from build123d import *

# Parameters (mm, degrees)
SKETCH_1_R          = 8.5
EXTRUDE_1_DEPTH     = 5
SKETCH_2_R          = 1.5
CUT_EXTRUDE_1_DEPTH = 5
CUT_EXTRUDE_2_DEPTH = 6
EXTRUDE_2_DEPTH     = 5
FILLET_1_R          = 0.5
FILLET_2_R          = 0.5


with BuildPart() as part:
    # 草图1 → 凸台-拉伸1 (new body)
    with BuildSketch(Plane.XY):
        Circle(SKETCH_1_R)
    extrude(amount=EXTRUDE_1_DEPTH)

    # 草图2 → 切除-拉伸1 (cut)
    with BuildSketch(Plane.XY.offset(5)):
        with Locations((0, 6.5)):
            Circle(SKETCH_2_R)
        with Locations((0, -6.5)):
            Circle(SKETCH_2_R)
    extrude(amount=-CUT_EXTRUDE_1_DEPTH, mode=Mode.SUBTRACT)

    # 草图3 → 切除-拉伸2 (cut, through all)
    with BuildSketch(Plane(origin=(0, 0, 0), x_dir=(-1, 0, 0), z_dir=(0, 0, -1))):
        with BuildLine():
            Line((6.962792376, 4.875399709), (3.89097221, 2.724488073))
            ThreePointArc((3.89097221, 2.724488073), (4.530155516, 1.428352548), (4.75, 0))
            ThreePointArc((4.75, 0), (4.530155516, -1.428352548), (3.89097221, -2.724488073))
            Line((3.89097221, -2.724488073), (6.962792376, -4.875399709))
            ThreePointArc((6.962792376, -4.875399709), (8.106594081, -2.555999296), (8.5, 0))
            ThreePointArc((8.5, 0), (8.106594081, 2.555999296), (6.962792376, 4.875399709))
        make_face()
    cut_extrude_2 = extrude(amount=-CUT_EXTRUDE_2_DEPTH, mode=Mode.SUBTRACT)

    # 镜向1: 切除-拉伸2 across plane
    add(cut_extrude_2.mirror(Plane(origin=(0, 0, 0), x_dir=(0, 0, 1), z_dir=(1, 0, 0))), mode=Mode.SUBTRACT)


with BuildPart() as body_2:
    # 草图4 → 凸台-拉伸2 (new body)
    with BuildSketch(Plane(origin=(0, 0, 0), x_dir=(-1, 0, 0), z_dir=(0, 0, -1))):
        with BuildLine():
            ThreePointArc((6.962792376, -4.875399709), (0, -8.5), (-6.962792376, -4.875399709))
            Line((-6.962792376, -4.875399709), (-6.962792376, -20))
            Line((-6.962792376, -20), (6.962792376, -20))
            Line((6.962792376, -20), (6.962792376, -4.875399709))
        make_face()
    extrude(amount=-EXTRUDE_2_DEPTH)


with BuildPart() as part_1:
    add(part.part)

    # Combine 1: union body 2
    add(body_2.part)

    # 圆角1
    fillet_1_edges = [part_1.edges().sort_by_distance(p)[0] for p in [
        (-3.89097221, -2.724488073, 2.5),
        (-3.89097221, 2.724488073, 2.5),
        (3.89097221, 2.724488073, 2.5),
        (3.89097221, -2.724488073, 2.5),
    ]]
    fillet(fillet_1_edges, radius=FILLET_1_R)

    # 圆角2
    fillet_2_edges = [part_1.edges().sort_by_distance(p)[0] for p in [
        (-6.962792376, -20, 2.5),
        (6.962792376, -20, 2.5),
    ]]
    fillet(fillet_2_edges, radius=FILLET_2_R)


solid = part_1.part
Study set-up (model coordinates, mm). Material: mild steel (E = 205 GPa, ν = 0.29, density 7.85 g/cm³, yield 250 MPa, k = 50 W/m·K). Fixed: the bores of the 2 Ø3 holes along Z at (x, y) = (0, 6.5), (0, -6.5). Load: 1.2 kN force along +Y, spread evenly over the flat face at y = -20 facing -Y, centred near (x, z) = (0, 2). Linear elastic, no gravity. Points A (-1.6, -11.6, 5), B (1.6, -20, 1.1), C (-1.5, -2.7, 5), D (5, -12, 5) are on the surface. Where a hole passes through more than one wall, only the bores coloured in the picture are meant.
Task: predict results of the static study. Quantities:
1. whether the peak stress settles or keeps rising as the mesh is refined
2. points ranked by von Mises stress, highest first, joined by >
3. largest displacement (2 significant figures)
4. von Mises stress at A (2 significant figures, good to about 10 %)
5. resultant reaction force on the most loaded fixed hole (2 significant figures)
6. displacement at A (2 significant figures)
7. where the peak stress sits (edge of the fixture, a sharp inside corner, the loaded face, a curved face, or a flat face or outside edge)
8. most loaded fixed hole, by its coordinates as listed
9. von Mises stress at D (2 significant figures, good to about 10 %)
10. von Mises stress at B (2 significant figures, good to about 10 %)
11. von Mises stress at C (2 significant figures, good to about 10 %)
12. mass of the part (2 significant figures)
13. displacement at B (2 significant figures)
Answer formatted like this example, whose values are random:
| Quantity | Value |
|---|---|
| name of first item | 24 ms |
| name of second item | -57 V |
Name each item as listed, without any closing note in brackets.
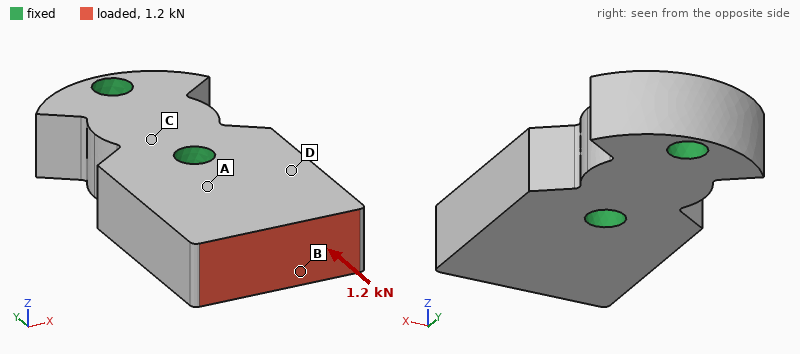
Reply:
| Quantity | Value |
|---|---|
| whether the peak stress settles or keeps rising as the mesh is refined | keeps rising |
| points ranked by von Mises stress, highest first, joined by > | A > B > D > C |
| largest displacement | 1.4 µm |
| von Mises stress at A | 24 MPa |
| resultant reaction force on the most loaded fixed hole | 1.1 kN |
| displacement at A | 0.60 µm |
| where the peak stress sits | edge of the fixture |
| most loaded fixed hole, by its coordinates as listed | (0, -6.5) |
| von Mises stress at D | 14 MPa |
| von Mises stress at B | 18 MPa |
| von Mises stress at C | 8.0 MPa |
| mass of the part | 13 g |
| displacement at B | 1.4 µm |
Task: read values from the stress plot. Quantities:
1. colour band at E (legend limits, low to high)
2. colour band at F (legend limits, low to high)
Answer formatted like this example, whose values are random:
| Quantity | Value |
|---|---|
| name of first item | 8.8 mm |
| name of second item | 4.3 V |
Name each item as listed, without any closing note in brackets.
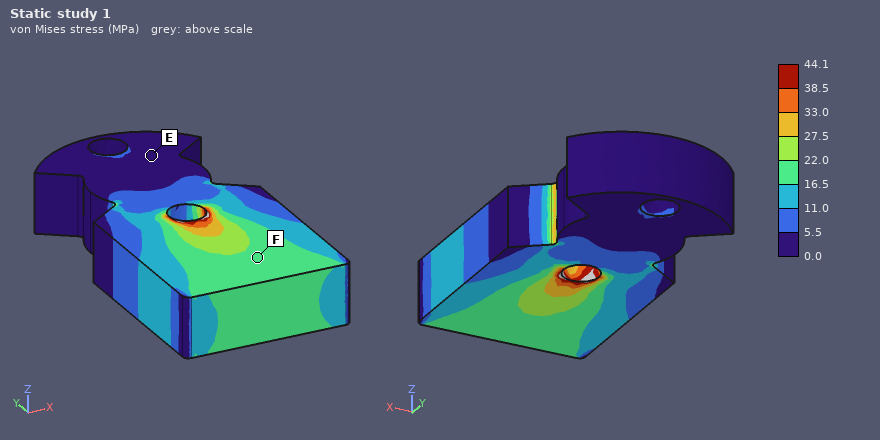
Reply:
| Quantity | Value |
|---|---|
| colour band at E | 0.0 to 5.5 MPa |
| colour band at F | 16.5 to 22.0 MPa |
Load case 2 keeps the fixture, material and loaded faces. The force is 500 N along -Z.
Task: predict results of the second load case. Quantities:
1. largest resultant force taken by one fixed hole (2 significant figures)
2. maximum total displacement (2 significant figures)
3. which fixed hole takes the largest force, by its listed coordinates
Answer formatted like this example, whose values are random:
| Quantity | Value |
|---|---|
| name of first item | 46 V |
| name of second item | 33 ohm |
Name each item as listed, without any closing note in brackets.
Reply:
| Quantity | Value |
|---|---|
| largest resultant force taken by one fixed hole | 600 N |
| maximum total displacement | 17 µm |
| which fixed hole takes the largest force, by its listed coordinates | (0, -6.5) |
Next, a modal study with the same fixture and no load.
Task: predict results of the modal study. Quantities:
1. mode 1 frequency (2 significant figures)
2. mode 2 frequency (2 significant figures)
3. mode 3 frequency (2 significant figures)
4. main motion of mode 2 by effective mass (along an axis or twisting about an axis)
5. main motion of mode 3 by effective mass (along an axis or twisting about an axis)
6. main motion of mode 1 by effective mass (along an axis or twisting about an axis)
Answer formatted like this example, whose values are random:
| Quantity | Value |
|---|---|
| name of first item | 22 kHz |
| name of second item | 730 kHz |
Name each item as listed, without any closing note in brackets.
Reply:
| Quantity | Value |
|---|---|
| mode 1 frequency | 20 kHz |
| mode 2 frequency | 25 kHz |
| mode 3 frequency | 34 kHz |
| main motion of mode 2 by effective mass | along X |
| main motion of mode 3 by effective mass | twisting about Y |
| main motion of mode 1 by effective mass | along Z |
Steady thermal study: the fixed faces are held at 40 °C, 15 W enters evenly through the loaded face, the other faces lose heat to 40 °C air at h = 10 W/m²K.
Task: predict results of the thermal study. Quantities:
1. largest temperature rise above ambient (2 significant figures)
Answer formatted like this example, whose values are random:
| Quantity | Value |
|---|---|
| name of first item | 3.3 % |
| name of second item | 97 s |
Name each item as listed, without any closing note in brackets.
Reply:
| Quantity | Value |
|---|---|
| largest temperature rise above ambient | 61 K |
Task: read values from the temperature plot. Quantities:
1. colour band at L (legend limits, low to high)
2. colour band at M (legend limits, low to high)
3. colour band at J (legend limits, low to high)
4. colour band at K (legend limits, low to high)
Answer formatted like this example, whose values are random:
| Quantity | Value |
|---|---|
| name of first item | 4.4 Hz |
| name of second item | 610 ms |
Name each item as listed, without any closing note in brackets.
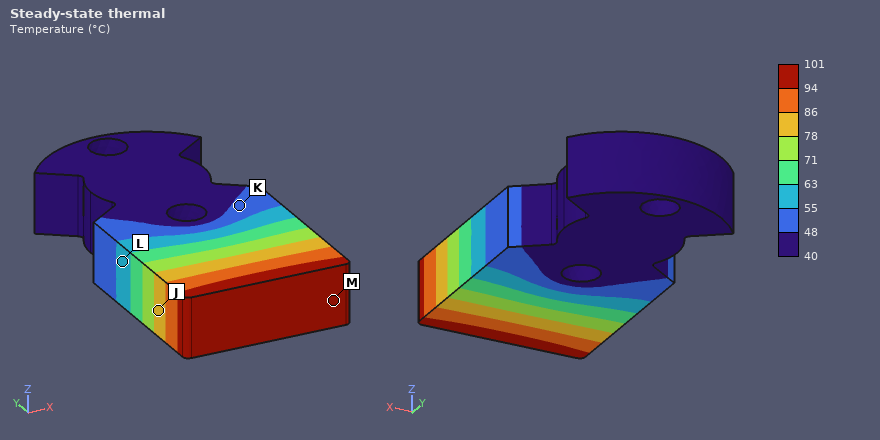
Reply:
| Quantity | Value |
|---|---|
| colour band at L | 55 to 63 °C |
| colour band at M | 94 to 101 °C |
| colour band at J | 78 to 86 °C |
| colour band at K | 48 to 55 °C |
